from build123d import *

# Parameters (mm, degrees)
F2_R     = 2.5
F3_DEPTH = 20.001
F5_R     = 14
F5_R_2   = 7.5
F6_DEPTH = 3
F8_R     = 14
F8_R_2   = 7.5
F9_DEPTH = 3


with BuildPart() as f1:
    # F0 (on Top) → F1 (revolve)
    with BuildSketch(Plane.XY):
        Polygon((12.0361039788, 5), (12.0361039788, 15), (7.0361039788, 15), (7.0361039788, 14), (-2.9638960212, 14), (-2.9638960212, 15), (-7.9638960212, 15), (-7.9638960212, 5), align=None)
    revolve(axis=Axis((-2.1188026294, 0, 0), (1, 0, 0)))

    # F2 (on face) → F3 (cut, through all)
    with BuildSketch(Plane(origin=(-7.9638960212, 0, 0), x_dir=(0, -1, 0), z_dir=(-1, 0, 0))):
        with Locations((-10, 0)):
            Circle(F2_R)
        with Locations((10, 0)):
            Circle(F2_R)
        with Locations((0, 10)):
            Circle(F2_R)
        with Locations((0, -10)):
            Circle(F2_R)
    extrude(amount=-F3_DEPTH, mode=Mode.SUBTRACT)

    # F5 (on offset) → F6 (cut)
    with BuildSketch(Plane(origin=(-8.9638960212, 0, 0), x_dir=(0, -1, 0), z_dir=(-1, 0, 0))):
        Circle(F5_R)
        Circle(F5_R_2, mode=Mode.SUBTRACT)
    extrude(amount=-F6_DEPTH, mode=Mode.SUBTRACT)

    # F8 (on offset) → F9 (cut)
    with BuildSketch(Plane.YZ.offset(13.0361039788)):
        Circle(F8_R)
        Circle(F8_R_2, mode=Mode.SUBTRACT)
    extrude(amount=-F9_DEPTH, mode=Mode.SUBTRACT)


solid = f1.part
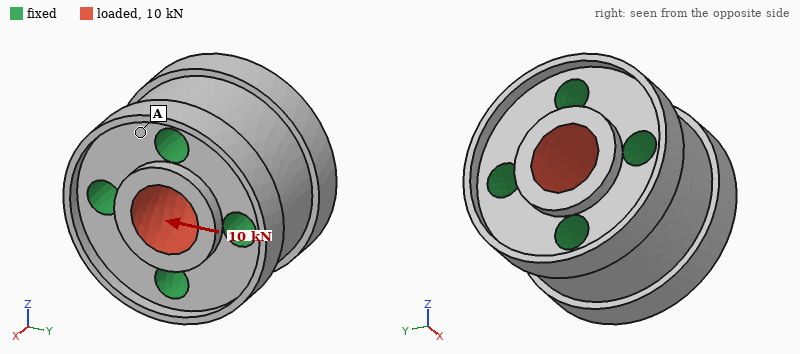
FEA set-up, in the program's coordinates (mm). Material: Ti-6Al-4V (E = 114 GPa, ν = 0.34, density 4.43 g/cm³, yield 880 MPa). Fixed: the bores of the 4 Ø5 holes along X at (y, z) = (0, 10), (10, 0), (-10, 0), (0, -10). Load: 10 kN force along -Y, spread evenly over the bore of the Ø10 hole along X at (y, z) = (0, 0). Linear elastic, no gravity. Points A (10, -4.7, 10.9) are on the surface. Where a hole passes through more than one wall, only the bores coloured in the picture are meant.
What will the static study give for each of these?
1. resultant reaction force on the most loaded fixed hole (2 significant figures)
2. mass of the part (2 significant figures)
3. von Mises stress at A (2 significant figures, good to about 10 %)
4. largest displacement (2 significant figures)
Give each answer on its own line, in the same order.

3.0 kN
38 g
7.0 MPa
2.1 µm
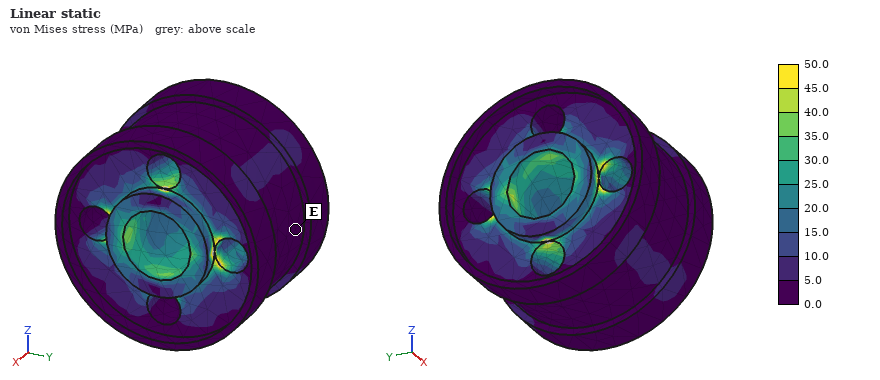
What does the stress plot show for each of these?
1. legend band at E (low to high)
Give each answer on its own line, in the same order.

0.0 to 5.0 MPa
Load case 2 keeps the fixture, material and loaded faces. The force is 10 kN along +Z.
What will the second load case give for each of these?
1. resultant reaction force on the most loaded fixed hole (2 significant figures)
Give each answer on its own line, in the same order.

3.0 kN
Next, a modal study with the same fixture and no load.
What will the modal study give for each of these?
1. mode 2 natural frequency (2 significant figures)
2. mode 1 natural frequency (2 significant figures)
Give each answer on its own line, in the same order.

91 kHz
88 kHz
